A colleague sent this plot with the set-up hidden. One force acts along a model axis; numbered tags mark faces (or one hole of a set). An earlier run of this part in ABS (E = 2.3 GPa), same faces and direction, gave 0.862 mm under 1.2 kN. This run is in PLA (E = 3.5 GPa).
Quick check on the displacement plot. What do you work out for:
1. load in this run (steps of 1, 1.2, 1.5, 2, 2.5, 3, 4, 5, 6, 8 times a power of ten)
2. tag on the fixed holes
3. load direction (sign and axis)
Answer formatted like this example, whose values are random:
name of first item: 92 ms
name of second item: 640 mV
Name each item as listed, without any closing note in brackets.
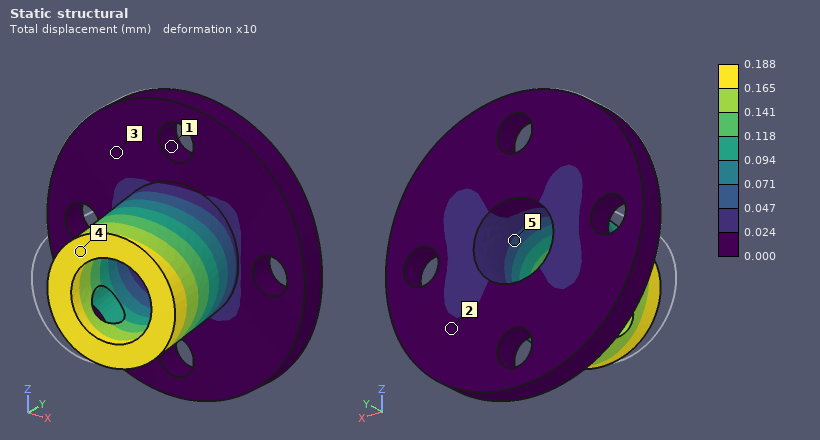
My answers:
load in this run: 400 N
tag on the fixed holes: 1
load direction: +X
